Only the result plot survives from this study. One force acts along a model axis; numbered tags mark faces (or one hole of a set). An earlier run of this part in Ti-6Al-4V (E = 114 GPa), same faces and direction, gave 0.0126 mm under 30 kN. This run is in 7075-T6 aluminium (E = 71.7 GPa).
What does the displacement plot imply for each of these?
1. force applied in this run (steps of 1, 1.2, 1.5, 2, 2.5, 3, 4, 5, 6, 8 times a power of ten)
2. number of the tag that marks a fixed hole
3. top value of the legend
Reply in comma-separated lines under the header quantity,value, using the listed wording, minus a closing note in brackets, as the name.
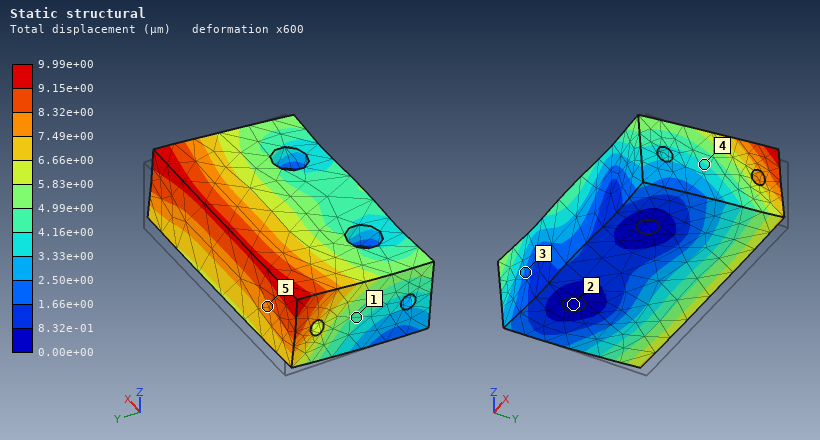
quantity,value
force applied in this run,15 kN
number of the tag that marks a fixed hole,2
top value of the legend,9.99e+00 µm
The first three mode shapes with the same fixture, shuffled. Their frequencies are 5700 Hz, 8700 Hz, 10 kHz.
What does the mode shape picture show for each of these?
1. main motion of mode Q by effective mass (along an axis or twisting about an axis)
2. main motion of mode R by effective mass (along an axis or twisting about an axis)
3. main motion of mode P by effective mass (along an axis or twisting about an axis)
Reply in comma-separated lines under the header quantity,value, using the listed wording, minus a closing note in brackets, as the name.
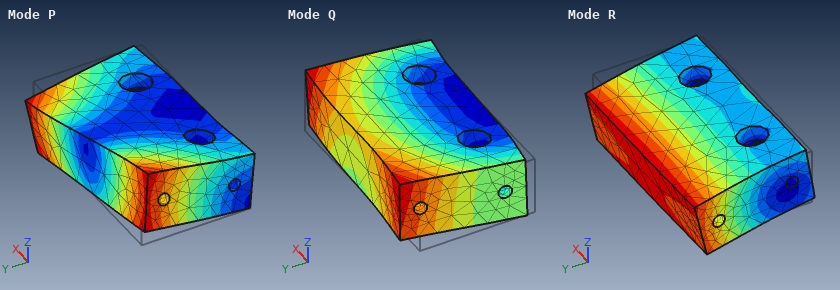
quantity,value
main motion of mode Q by effective mass,along X
main motion of mode R by effective mass,along Z
main motion of mode P by effective mass,twisting about Y
